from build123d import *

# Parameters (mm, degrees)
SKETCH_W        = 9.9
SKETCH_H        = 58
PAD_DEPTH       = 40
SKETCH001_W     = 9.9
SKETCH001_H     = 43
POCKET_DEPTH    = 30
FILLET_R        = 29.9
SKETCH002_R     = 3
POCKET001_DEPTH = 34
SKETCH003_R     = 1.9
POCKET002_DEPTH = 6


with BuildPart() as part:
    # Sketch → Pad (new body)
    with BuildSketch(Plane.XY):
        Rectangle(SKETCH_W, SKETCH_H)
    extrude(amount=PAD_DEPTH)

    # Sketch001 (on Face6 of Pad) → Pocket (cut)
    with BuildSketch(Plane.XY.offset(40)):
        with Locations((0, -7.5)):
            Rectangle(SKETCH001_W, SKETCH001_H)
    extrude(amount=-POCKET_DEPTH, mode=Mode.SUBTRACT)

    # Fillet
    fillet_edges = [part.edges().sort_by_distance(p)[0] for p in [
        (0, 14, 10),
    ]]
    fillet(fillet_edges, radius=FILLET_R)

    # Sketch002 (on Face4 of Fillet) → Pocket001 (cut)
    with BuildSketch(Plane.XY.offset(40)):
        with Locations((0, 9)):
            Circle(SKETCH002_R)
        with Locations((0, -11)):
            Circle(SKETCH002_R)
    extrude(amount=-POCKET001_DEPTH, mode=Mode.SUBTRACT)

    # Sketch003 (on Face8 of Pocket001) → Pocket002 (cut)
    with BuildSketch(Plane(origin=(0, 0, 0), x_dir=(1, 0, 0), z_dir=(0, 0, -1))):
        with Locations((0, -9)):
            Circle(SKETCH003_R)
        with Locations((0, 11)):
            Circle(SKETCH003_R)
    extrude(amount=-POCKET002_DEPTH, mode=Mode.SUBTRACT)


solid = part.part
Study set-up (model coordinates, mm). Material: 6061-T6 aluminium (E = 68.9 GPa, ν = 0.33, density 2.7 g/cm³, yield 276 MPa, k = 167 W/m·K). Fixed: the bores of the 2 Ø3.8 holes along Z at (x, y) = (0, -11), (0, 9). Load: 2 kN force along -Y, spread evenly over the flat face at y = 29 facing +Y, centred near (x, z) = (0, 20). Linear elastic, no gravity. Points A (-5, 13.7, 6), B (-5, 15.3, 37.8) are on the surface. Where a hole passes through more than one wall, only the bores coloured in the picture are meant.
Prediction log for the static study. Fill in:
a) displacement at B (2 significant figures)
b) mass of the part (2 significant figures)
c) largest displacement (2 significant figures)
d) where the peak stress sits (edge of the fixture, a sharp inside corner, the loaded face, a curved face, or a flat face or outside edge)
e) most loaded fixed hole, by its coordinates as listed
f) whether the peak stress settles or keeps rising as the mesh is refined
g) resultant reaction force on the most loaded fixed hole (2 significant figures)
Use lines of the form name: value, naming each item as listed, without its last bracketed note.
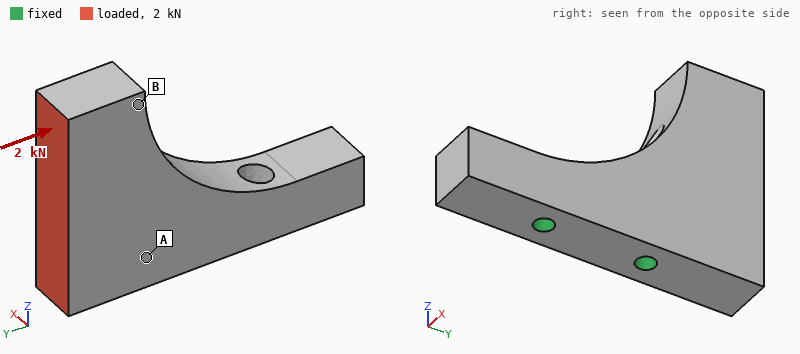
displacement at B: 59 µm
mass of the part: 31 g
largest displacement: 71 µm
where the peak stress sits: edge of the fixture
most loaded fixed hole, by its coordinates as listed: (0, -11)
whether the peak stress settles or keeps rising as the mesh is refined: keeps rising
resultant reaction force on the most loaded fixed hole: 1.9 kN
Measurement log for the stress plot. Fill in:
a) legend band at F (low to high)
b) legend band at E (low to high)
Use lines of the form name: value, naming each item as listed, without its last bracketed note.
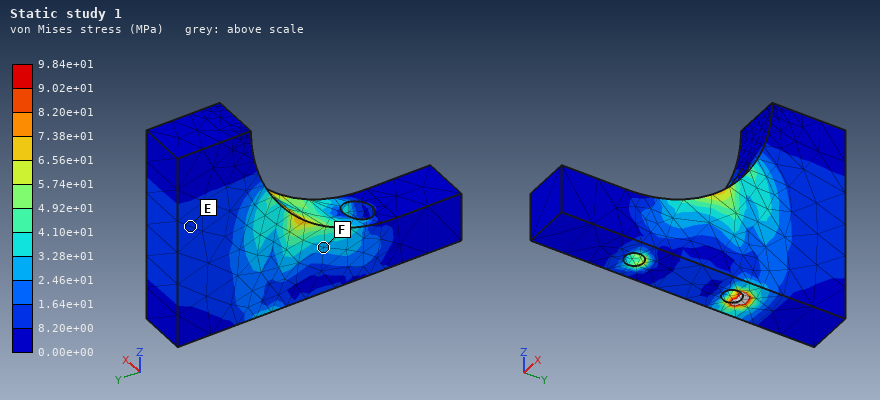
legend band at F: 2.46e+01 to 3.28e+01 MPa
legend band at E: 8.20e+00 to 1.64e+01 MPa
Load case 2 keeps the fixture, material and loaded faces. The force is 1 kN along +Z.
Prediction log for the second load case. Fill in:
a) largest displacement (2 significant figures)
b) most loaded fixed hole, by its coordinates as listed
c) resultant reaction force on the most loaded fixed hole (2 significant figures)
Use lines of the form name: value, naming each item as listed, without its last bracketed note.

largest displacement: 48 µm
most loaded fixed hole, by its coordinates as listed: (0, 9)
resultant reaction force on the most loaded fixed hole: 1.8 kN
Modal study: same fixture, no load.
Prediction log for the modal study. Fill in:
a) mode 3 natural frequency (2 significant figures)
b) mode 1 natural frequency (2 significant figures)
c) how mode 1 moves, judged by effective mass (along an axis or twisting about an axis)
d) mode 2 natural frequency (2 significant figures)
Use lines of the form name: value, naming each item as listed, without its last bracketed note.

mode 3 natural frequency: 12 kHz
mode 1 natural frequency: 4000 Hz
how mode 1 moves, judged by effective mass: along X
mode 2 natural frequency: 7000 Hz
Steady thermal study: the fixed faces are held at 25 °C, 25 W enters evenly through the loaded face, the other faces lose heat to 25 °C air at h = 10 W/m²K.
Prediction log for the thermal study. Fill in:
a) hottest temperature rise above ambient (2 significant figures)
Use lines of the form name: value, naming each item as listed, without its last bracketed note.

hottest temperature rise above ambient: 22 K
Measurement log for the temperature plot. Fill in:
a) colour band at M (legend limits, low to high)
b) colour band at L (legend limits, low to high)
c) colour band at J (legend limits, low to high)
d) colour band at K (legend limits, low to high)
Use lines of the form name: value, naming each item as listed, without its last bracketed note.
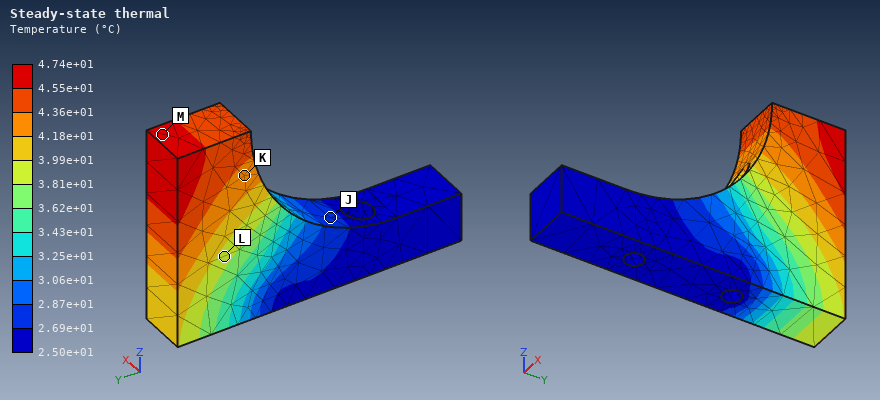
colour band at M: 4.55e+01 to 4.74e+01 °C
colour band at L: 3.81e+01 to 3.99e+01 °C
colour band at J: 2.69e+01 to 2.87e+01 °C
colour band at K: 4.18e+01 to 4.36e+01 °C
